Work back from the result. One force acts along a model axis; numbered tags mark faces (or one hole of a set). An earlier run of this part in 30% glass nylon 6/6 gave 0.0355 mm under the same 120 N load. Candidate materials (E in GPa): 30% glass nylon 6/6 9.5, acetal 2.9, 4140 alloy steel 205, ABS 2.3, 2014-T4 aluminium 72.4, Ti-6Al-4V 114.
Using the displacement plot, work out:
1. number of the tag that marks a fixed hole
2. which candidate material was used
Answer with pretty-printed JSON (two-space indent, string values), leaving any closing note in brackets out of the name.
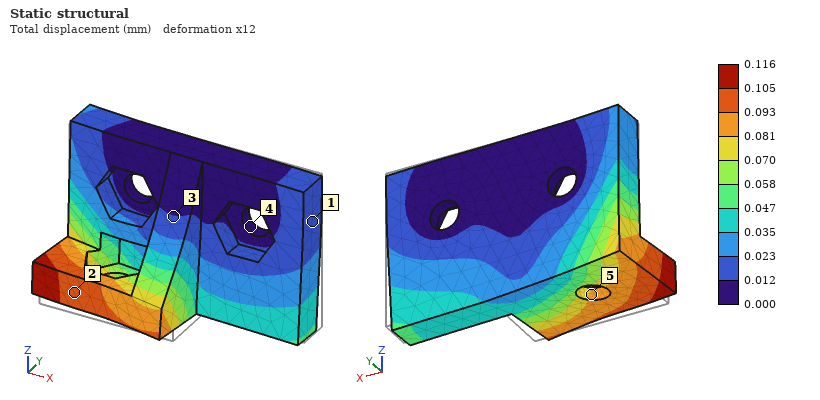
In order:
{
  "number of the tag that marks a fixed hole": "4",
  "which candidate material was used": "acetal"
}
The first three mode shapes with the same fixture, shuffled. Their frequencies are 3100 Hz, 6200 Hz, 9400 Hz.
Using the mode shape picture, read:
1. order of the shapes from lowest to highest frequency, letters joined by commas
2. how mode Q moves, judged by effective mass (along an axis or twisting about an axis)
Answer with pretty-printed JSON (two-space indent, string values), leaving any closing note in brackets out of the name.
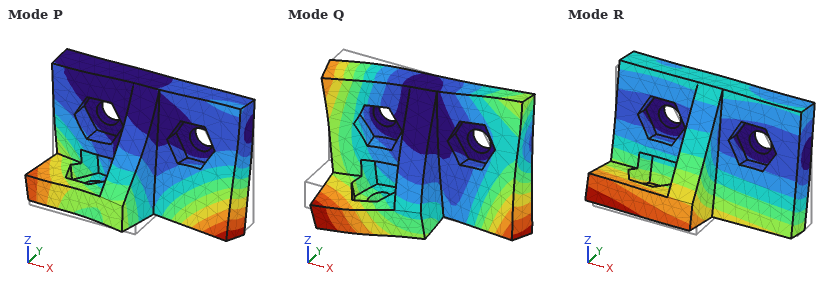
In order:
{
  "order of the shapes from lowest to highest frequency, letters joined by commas": "R, P, Q",
  "how mode Q moves, judged by effective mass": "along X"
}
